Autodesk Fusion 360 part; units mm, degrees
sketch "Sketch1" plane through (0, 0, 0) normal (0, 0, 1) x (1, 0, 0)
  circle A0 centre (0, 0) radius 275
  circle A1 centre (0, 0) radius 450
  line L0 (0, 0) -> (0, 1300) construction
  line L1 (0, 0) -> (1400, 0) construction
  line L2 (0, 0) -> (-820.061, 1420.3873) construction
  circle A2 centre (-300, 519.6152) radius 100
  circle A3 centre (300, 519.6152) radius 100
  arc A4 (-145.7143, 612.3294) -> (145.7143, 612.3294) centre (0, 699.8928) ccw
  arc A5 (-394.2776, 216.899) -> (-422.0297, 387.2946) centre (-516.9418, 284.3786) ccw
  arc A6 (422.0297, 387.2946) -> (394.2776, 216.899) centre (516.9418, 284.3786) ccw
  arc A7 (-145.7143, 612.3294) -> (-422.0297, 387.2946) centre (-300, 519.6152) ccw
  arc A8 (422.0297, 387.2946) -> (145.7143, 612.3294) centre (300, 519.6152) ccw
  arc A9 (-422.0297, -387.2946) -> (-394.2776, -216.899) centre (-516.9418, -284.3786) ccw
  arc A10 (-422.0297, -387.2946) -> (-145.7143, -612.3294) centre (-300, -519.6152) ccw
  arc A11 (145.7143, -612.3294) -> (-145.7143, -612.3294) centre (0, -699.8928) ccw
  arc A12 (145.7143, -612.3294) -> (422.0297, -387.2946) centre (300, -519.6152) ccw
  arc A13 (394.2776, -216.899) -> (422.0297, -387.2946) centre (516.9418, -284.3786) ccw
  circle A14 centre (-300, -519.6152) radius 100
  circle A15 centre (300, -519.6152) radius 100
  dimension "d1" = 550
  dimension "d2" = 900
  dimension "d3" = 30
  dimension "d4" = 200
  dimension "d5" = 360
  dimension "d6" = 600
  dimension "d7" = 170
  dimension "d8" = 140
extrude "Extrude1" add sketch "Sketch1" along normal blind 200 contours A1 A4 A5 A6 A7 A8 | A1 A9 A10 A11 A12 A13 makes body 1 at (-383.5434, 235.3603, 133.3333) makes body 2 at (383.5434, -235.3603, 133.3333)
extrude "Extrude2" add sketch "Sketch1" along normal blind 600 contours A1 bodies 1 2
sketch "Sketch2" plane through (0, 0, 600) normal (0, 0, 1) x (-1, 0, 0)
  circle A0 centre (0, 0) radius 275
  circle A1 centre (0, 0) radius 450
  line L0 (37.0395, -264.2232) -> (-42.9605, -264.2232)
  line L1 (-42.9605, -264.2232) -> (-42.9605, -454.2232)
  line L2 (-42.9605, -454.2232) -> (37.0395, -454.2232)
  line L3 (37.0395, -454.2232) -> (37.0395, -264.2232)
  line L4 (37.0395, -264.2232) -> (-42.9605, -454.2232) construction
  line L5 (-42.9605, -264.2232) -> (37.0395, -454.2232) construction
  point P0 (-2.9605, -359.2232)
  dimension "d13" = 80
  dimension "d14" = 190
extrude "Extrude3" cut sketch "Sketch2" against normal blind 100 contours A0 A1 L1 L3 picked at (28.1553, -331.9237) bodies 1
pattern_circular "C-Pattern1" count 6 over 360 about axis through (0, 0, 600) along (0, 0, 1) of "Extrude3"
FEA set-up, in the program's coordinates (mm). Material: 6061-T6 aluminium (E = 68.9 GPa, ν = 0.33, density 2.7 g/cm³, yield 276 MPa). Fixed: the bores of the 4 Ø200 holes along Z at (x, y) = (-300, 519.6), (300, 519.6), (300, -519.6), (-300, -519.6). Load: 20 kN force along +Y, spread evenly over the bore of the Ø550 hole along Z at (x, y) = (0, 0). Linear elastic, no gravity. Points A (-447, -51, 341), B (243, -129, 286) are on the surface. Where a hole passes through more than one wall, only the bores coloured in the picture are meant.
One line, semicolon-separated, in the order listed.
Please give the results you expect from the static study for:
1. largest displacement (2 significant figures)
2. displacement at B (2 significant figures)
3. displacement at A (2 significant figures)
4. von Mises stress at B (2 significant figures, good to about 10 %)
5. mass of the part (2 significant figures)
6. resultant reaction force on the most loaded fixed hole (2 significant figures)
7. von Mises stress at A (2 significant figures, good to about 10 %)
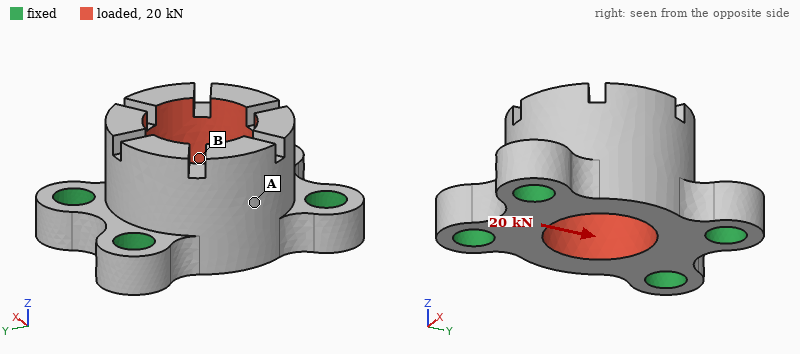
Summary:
1.4 µm; 0.53 µm; 0.55 µm; 0.097 MPa; 810 kg; 5.5 kN; 0.026 MPa
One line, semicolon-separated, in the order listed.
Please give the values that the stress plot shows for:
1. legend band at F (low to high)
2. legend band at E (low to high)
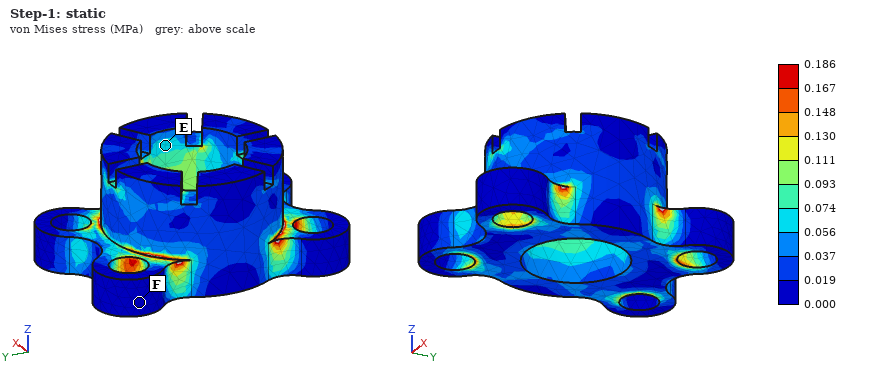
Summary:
0.000 to 0.019 MPa; 0.056 to 0.074 MPa
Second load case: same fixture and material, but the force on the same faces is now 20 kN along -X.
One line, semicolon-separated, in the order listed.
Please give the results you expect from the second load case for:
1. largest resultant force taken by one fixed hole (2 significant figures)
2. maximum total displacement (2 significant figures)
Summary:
6.3 kN; 2.5 µm
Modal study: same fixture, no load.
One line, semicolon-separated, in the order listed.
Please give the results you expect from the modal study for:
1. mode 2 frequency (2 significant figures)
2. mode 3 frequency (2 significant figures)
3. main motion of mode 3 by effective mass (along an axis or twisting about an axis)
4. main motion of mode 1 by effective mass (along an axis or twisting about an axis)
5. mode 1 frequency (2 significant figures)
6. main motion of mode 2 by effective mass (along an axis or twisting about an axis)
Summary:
770 Hz; 1000 Hz; along Y; along X; 670 Hz; along Z
